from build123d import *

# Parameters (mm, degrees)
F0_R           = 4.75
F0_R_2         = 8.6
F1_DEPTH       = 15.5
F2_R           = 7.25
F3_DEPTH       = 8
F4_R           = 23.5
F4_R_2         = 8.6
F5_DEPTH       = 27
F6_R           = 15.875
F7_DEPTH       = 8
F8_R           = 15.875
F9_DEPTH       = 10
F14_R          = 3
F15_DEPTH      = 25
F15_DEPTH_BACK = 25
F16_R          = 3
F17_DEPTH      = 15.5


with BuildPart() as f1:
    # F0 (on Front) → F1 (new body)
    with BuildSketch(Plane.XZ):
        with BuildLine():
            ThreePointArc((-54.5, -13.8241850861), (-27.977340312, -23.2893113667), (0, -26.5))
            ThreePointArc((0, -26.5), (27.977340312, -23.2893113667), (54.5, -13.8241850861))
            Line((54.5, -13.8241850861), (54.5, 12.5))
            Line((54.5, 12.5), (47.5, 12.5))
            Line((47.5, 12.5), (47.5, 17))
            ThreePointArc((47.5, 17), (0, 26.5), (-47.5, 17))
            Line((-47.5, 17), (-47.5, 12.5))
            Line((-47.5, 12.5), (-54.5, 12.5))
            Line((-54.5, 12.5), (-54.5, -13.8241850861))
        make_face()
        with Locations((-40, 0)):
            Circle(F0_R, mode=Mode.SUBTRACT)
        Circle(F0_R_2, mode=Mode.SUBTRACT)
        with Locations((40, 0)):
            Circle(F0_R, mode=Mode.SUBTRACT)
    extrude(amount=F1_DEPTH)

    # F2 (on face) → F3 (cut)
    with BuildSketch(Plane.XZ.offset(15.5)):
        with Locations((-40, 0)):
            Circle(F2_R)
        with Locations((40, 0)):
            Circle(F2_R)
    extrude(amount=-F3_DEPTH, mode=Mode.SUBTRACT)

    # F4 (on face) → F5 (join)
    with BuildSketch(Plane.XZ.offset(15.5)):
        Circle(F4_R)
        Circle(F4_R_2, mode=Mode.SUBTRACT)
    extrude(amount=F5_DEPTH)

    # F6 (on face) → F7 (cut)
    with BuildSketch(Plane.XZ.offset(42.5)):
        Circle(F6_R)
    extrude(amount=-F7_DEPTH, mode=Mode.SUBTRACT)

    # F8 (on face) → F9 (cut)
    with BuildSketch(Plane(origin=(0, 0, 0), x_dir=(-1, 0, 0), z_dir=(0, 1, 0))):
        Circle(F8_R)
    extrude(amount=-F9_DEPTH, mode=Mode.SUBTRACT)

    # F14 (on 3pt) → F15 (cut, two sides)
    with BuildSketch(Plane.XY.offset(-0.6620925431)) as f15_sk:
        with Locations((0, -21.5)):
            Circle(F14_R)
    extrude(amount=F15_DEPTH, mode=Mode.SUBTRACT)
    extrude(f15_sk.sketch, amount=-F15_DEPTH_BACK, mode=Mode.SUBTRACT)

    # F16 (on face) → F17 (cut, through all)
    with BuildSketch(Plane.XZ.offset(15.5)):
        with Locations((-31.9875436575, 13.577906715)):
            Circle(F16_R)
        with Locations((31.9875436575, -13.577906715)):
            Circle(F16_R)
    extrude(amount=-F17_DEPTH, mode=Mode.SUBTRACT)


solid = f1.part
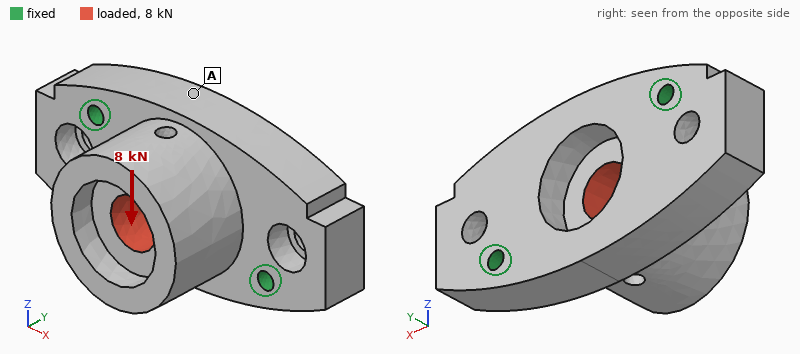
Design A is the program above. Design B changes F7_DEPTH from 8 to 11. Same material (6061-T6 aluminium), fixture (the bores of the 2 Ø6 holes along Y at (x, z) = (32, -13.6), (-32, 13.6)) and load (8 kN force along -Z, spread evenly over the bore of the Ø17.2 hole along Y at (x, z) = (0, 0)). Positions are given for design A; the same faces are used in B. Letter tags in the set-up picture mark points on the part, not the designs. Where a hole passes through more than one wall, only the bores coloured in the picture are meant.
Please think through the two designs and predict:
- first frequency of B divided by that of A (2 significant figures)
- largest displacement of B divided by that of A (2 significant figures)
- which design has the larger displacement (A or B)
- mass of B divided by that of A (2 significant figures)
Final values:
1.0
0.89
A
0.98
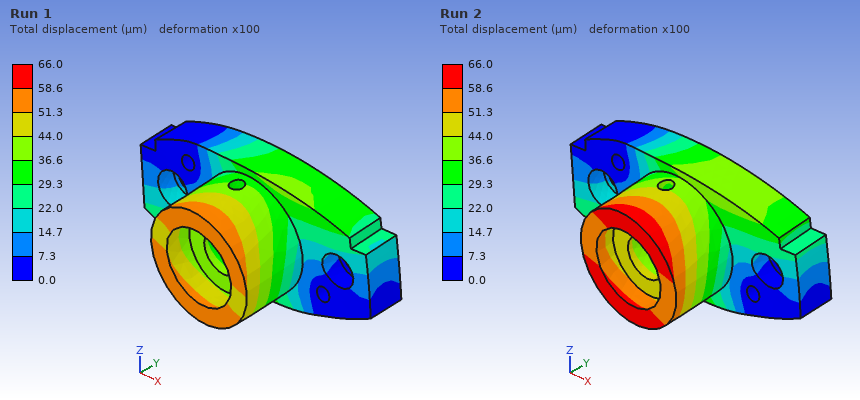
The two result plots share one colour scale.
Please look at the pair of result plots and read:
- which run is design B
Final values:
Run 1
